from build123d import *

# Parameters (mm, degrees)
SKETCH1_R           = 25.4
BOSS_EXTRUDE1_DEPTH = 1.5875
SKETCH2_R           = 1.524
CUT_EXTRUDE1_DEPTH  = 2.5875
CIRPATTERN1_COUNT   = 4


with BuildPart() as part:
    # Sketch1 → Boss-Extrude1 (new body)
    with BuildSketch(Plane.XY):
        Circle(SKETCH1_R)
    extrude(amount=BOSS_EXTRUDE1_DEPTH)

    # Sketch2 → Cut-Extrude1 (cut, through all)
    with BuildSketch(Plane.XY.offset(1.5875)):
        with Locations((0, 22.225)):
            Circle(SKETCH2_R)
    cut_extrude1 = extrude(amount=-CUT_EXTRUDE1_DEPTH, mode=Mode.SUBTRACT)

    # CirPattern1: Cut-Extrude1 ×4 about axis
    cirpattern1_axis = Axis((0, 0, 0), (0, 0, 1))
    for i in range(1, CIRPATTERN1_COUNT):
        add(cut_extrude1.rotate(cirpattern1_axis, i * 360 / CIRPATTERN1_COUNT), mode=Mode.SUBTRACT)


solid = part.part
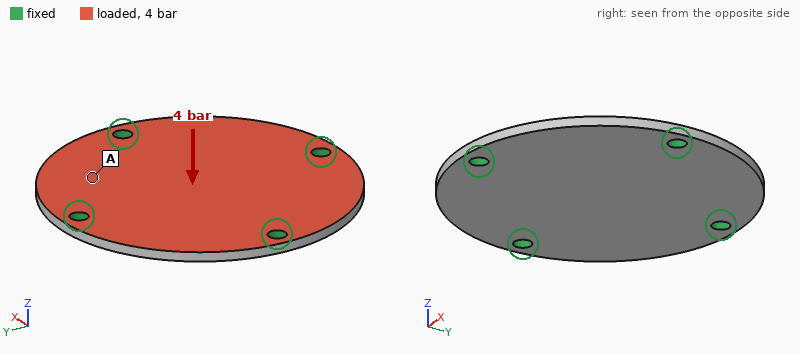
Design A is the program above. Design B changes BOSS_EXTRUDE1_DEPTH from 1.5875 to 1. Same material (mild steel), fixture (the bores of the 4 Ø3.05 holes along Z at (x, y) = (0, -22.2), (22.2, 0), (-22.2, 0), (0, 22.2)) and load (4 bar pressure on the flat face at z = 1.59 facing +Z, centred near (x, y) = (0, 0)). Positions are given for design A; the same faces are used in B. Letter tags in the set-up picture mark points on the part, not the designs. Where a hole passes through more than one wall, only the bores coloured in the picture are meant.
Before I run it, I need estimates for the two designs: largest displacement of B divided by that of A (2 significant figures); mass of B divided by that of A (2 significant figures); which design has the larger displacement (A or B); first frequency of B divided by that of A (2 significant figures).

3.8
0.63
B
0.65
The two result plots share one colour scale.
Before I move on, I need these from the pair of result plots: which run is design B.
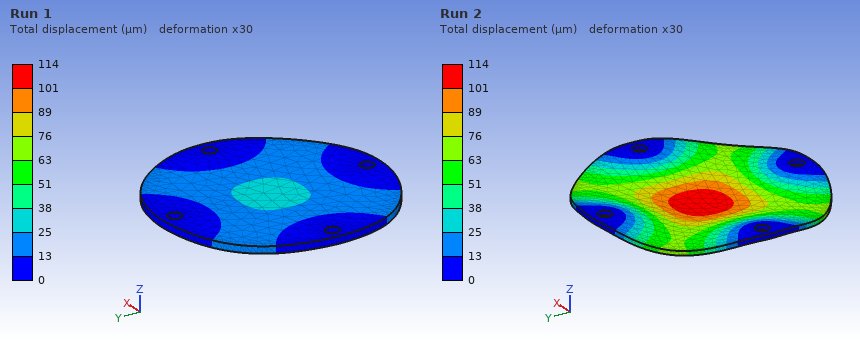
Run 2
